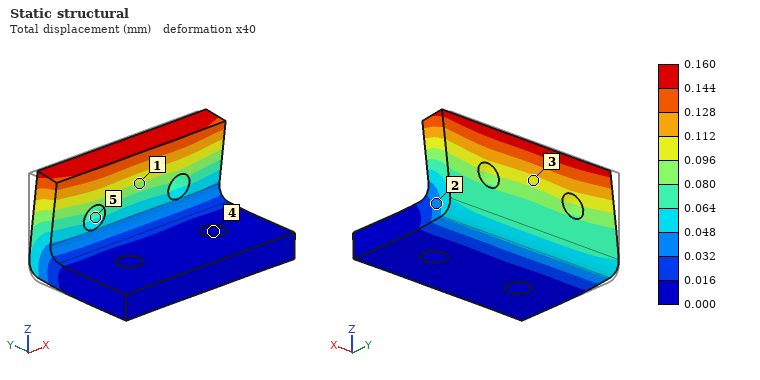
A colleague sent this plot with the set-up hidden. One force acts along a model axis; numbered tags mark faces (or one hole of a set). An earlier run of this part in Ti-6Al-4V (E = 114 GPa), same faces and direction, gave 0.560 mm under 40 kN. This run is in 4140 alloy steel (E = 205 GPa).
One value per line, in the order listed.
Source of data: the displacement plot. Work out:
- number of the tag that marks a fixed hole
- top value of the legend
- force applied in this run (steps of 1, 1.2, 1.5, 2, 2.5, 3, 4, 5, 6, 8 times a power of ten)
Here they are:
4
0.160 mm
20 kN
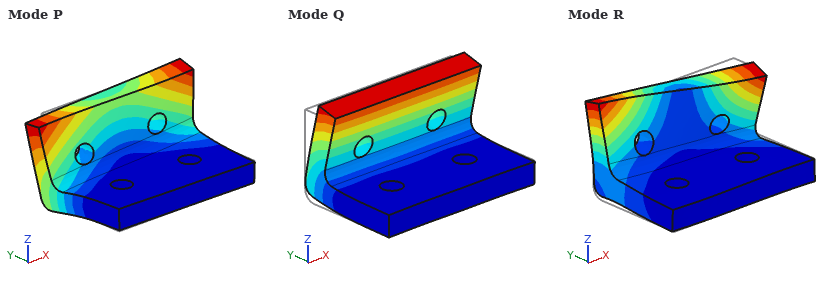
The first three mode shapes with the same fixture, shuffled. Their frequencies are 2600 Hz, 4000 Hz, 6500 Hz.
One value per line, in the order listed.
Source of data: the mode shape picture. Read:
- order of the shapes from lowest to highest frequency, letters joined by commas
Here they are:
Q, P, R
